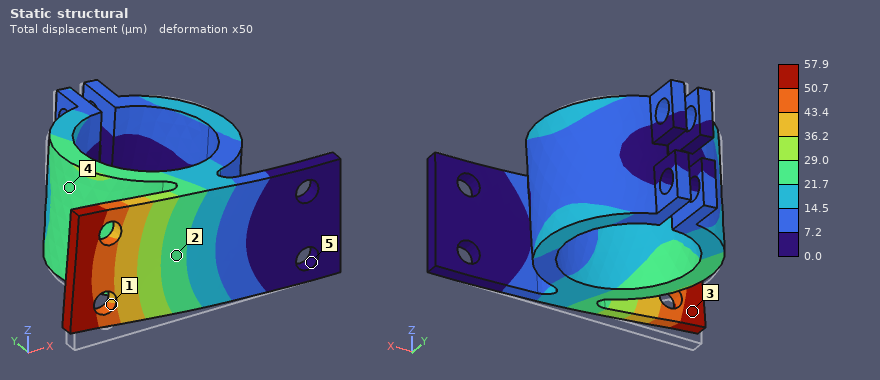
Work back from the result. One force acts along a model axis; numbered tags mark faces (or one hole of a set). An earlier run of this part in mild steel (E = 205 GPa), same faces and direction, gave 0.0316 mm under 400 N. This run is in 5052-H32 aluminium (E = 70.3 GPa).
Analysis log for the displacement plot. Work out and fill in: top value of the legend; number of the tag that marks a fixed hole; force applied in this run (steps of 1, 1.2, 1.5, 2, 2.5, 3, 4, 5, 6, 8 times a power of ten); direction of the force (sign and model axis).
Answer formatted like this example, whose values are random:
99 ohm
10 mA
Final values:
57.9 µm
5
250 N
+Z
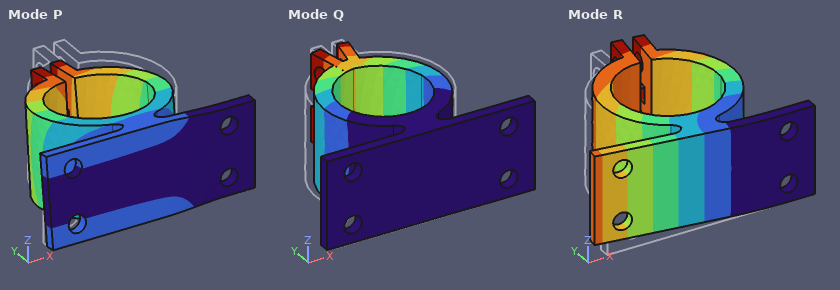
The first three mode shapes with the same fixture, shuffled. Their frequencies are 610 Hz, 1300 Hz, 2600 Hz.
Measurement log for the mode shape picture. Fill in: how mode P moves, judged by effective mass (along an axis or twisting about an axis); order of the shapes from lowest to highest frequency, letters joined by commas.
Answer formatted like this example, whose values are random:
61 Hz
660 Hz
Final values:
along Z
R, P, Q
